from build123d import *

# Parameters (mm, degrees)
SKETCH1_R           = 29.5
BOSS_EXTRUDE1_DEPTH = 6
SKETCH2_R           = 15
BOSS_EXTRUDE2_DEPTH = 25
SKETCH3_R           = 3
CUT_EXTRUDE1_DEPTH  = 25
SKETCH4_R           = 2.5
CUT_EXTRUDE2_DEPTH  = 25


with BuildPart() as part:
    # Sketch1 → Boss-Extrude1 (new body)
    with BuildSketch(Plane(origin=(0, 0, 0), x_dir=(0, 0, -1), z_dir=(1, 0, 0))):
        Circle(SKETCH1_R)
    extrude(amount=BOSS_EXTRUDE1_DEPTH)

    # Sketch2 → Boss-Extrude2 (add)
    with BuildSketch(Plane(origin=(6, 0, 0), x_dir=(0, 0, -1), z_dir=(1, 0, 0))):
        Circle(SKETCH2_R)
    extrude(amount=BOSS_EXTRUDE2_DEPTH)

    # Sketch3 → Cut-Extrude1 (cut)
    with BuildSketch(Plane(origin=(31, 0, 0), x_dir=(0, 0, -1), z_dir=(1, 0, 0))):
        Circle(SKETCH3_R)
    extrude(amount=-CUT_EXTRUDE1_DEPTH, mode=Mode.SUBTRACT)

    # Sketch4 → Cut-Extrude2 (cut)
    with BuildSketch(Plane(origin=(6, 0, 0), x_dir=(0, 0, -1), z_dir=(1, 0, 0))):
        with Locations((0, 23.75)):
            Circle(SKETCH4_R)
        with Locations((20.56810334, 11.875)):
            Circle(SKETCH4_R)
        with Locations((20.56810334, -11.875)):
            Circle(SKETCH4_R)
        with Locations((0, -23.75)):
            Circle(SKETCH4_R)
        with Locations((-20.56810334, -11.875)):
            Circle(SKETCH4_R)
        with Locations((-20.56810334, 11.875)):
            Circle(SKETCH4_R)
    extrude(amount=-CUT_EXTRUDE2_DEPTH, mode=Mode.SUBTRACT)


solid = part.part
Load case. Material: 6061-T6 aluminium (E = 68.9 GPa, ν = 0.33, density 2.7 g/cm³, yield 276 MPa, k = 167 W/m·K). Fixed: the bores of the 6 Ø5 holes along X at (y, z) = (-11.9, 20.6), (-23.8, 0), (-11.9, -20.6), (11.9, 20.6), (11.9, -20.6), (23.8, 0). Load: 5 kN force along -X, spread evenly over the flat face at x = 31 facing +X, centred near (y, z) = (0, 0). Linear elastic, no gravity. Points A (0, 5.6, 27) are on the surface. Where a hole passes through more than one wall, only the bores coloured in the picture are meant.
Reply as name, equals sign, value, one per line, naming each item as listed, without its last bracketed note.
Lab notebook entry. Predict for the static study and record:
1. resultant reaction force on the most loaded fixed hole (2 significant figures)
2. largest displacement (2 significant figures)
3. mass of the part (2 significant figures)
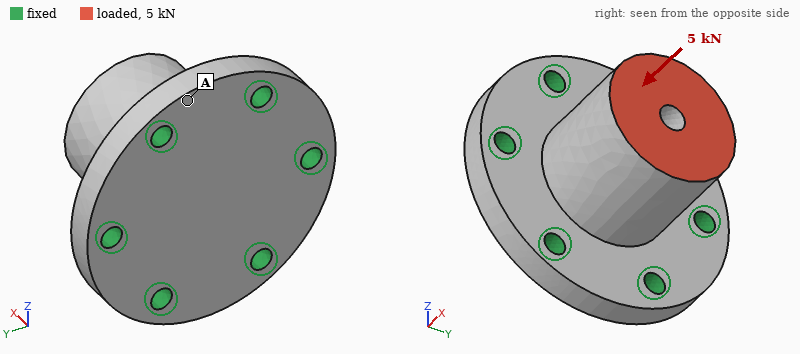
resultant reaction force on the most loaded fixed hole = 890 N
largest displacement = 11 µm
mass of the part = 88 g
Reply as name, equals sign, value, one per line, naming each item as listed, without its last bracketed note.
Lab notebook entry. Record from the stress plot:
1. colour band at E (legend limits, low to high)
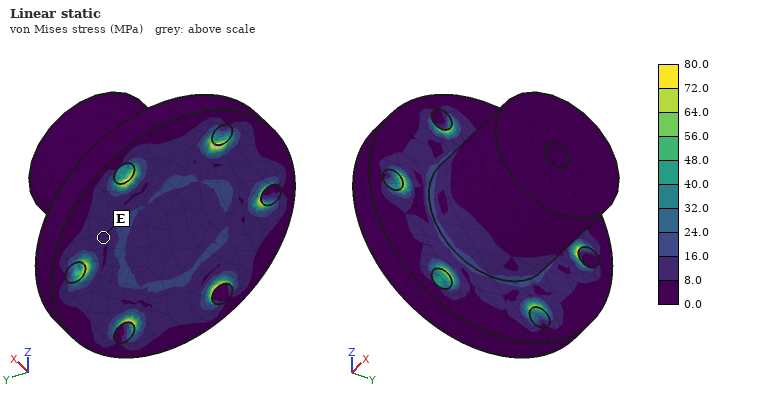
colour band at E = 8.0 to 16.0 MPa
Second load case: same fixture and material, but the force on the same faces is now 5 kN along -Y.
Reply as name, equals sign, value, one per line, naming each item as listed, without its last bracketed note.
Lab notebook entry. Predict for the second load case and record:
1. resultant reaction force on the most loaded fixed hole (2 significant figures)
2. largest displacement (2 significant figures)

resultant reaction force on the most loaded fixed hole = 2.7 kN
largest displacement = 59 µm
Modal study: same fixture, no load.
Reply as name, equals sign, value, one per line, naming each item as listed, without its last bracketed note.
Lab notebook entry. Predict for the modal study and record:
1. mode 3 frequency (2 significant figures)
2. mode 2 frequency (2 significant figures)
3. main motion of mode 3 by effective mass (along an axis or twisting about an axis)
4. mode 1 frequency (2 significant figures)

mode 3 frequency = 15 kHz
mode 2 frequency = 11 kHz
main motion of mode 3 by effective mass = along X
mode 1 frequency = 11 kHz
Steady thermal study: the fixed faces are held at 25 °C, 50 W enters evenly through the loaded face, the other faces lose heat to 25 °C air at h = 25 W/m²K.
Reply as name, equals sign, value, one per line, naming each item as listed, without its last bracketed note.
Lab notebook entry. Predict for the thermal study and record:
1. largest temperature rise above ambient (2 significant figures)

largest temperature rise above ambient = 17 K
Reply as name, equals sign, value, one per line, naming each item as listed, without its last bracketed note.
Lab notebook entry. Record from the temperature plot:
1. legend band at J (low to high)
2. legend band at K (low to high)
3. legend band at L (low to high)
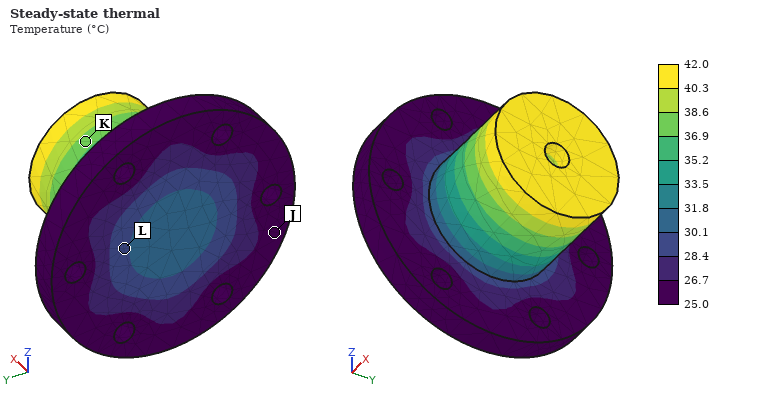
legend band at J = 25.0 to 26.7 °C
legend band at K = 36.9 to 38.6 °C
legend band at L = 28.4 to 30.1 °C
